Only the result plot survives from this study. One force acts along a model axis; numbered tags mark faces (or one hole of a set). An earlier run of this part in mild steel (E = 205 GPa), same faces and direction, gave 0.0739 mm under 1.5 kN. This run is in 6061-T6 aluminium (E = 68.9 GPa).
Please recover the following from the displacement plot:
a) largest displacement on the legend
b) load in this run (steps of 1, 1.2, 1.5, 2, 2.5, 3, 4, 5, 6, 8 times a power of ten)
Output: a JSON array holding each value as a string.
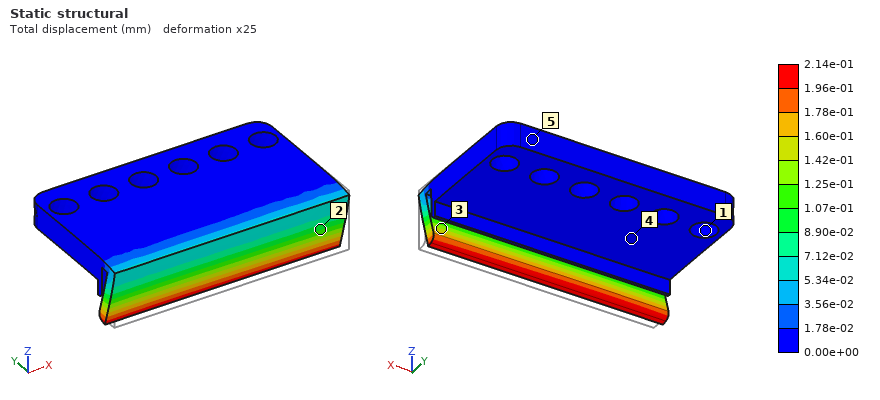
["2.14e-01 mm", "1.5 kN"]
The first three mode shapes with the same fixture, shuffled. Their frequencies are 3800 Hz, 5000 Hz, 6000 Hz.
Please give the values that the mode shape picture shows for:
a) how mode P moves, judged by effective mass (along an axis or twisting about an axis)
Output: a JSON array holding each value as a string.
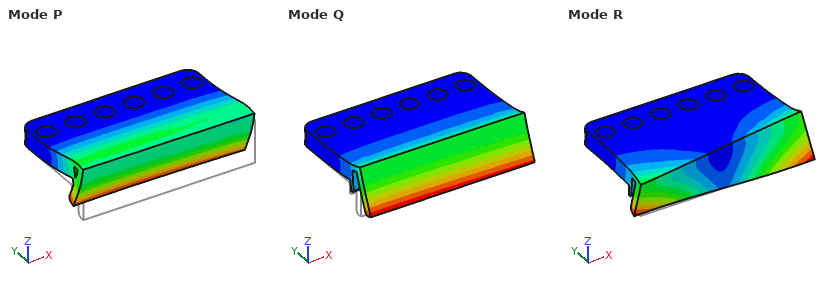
["along Z"]
